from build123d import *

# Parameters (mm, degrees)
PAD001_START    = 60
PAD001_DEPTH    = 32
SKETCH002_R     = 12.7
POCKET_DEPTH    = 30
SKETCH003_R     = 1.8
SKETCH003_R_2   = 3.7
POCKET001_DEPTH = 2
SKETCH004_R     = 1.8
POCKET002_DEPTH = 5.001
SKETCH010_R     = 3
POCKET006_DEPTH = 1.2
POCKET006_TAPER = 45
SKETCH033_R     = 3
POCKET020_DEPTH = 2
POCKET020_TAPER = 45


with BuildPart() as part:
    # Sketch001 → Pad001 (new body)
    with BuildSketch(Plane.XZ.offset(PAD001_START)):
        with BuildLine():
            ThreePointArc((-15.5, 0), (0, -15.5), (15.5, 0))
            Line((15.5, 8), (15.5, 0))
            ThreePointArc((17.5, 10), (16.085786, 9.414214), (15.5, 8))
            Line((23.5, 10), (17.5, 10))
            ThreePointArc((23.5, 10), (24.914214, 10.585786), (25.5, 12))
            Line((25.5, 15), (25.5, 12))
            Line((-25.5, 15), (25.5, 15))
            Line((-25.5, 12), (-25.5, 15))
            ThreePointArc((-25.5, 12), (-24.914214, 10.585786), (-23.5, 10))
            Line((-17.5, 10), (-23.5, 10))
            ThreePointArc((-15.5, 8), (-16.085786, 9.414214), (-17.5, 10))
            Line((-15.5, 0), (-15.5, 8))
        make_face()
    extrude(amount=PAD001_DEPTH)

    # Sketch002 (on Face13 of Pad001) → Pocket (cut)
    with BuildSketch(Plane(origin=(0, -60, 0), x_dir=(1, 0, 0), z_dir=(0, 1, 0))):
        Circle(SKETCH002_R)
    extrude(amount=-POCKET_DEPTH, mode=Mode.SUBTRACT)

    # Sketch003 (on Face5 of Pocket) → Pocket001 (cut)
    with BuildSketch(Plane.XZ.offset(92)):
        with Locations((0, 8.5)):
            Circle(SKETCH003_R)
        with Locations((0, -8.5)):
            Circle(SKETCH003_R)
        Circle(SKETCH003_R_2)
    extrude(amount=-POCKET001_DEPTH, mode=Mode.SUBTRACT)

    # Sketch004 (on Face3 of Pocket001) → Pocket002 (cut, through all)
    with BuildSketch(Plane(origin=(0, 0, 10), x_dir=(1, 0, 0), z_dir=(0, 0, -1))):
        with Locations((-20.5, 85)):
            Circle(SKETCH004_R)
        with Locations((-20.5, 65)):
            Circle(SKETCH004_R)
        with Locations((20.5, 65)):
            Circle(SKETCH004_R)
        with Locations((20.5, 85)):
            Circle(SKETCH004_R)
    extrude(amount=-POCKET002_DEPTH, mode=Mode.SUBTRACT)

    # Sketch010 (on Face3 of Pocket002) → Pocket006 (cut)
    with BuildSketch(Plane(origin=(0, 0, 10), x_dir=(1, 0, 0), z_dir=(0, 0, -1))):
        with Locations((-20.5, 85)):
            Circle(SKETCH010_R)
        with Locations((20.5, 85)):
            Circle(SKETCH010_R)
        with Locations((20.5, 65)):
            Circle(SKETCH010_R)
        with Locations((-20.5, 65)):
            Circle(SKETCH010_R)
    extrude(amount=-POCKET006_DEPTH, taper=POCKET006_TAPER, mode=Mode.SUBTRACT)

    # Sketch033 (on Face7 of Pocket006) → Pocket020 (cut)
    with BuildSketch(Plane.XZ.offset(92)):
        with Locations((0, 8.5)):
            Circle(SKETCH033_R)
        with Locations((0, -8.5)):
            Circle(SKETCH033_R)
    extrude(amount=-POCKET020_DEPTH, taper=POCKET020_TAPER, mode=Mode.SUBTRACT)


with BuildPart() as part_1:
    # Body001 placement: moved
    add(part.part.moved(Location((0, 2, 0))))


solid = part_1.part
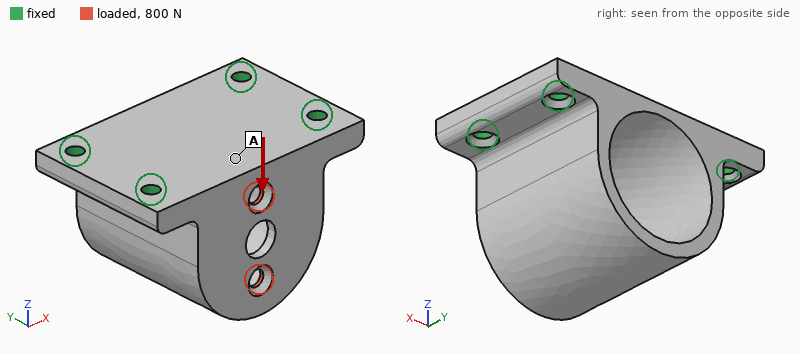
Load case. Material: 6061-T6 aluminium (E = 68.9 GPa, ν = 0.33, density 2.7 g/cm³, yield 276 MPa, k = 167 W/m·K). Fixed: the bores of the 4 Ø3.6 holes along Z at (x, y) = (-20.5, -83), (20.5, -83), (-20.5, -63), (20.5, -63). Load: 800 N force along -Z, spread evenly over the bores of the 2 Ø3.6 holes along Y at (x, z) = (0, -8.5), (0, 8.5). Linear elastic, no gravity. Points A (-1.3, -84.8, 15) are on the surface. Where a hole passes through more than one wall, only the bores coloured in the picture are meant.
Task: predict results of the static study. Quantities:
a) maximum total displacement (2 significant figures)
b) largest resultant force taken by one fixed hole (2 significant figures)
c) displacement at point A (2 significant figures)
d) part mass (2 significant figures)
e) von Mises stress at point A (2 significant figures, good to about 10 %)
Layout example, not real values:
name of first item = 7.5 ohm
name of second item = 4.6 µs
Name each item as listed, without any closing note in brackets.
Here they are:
maximum total displacement = 14 µm
largest resultant force taken by one fixed hole = 510 N
displacement at point A = 8.5 µm
part mass = 39 g
von Mises stress at point A = 9.9 MPa
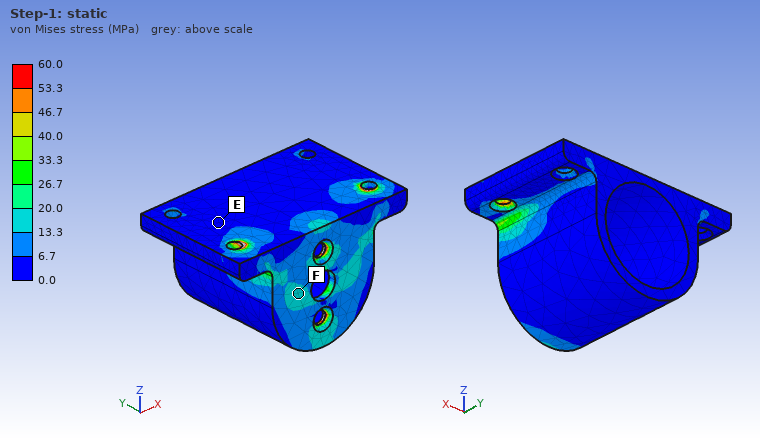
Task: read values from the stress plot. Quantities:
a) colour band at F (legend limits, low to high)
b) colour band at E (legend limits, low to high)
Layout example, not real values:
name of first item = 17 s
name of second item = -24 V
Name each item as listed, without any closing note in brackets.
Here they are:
colour band at F = 13.3 to 20.0 MPa
colour band at E = 0.0 to 6.7 MPa
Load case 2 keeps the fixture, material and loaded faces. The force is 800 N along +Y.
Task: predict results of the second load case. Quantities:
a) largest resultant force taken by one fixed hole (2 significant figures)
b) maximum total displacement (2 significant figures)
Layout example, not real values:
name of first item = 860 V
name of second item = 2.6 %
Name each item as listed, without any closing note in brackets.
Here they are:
largest resultant force taken by one fixed hole = 360 N
maximum total displacement = 39 µm
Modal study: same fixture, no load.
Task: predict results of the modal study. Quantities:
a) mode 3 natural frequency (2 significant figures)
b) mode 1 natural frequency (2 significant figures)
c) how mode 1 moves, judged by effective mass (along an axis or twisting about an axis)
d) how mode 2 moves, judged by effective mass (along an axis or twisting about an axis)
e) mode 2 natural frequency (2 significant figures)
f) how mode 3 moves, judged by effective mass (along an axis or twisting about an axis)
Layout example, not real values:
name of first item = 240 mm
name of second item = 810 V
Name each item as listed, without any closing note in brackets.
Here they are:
mode 3 natural frequency = 13 kHz
mode 1 natural frequency = 8400 Hz
how mode 1 moves, judged by effective mass = along X
how mode 2 moves, judged by effective mass = along Y
mode 2 natural frequency = 9700 Hz
how mode 3 moves, judged by effective mass = along Z
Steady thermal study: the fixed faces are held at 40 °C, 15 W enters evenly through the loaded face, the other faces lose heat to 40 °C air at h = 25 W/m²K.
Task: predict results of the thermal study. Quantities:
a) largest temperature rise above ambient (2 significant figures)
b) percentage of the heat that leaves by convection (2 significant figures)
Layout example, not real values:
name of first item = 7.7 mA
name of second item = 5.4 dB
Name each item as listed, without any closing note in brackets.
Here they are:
largest temperature rise above ambient = 17 K
percentage of the heat that leaves by convection = 5.8 %
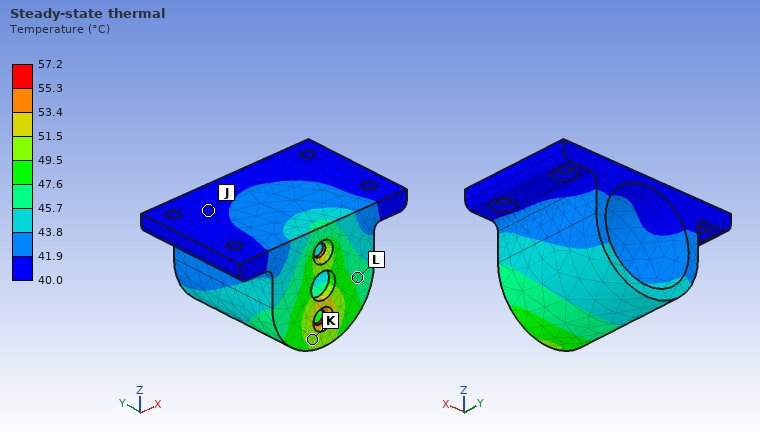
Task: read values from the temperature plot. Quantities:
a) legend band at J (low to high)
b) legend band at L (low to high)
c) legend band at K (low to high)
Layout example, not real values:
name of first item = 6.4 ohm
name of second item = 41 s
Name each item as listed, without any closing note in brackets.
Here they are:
legend band at J = 40.0 to 41.9 °C
legend band at L = 45.7 to 47.6 °C
legend band at K = 49.5 to 51.5 °C
